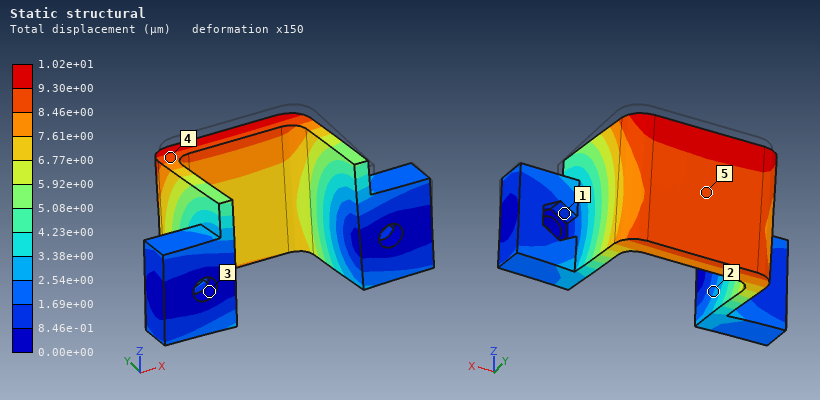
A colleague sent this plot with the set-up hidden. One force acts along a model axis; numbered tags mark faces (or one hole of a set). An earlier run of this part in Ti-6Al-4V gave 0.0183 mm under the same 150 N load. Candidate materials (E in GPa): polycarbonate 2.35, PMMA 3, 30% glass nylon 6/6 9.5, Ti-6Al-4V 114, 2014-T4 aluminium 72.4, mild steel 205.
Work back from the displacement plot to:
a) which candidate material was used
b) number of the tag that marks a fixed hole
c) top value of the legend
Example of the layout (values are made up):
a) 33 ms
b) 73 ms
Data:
a) mild steel
b) 3
c) 1.02e+01 µm
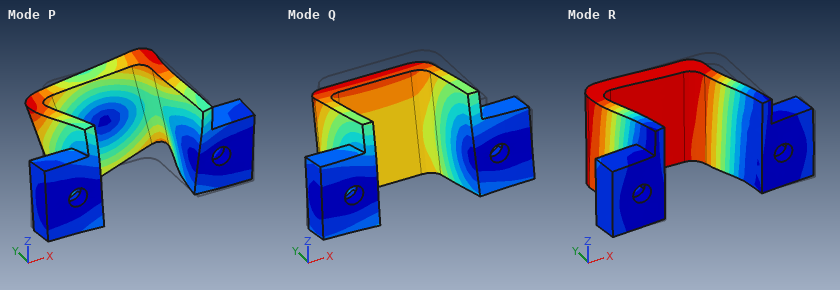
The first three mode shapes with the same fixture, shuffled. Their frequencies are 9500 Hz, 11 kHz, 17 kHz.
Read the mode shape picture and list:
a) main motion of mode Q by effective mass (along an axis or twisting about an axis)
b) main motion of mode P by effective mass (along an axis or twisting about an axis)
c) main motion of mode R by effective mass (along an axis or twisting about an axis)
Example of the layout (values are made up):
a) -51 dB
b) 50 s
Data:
a) along Z
b) twisting about Y
c) along X
